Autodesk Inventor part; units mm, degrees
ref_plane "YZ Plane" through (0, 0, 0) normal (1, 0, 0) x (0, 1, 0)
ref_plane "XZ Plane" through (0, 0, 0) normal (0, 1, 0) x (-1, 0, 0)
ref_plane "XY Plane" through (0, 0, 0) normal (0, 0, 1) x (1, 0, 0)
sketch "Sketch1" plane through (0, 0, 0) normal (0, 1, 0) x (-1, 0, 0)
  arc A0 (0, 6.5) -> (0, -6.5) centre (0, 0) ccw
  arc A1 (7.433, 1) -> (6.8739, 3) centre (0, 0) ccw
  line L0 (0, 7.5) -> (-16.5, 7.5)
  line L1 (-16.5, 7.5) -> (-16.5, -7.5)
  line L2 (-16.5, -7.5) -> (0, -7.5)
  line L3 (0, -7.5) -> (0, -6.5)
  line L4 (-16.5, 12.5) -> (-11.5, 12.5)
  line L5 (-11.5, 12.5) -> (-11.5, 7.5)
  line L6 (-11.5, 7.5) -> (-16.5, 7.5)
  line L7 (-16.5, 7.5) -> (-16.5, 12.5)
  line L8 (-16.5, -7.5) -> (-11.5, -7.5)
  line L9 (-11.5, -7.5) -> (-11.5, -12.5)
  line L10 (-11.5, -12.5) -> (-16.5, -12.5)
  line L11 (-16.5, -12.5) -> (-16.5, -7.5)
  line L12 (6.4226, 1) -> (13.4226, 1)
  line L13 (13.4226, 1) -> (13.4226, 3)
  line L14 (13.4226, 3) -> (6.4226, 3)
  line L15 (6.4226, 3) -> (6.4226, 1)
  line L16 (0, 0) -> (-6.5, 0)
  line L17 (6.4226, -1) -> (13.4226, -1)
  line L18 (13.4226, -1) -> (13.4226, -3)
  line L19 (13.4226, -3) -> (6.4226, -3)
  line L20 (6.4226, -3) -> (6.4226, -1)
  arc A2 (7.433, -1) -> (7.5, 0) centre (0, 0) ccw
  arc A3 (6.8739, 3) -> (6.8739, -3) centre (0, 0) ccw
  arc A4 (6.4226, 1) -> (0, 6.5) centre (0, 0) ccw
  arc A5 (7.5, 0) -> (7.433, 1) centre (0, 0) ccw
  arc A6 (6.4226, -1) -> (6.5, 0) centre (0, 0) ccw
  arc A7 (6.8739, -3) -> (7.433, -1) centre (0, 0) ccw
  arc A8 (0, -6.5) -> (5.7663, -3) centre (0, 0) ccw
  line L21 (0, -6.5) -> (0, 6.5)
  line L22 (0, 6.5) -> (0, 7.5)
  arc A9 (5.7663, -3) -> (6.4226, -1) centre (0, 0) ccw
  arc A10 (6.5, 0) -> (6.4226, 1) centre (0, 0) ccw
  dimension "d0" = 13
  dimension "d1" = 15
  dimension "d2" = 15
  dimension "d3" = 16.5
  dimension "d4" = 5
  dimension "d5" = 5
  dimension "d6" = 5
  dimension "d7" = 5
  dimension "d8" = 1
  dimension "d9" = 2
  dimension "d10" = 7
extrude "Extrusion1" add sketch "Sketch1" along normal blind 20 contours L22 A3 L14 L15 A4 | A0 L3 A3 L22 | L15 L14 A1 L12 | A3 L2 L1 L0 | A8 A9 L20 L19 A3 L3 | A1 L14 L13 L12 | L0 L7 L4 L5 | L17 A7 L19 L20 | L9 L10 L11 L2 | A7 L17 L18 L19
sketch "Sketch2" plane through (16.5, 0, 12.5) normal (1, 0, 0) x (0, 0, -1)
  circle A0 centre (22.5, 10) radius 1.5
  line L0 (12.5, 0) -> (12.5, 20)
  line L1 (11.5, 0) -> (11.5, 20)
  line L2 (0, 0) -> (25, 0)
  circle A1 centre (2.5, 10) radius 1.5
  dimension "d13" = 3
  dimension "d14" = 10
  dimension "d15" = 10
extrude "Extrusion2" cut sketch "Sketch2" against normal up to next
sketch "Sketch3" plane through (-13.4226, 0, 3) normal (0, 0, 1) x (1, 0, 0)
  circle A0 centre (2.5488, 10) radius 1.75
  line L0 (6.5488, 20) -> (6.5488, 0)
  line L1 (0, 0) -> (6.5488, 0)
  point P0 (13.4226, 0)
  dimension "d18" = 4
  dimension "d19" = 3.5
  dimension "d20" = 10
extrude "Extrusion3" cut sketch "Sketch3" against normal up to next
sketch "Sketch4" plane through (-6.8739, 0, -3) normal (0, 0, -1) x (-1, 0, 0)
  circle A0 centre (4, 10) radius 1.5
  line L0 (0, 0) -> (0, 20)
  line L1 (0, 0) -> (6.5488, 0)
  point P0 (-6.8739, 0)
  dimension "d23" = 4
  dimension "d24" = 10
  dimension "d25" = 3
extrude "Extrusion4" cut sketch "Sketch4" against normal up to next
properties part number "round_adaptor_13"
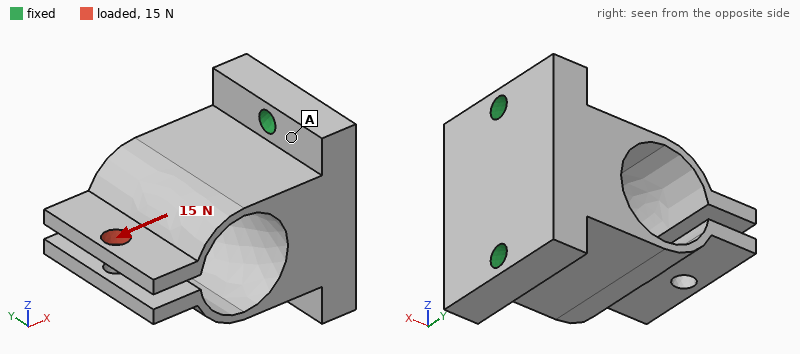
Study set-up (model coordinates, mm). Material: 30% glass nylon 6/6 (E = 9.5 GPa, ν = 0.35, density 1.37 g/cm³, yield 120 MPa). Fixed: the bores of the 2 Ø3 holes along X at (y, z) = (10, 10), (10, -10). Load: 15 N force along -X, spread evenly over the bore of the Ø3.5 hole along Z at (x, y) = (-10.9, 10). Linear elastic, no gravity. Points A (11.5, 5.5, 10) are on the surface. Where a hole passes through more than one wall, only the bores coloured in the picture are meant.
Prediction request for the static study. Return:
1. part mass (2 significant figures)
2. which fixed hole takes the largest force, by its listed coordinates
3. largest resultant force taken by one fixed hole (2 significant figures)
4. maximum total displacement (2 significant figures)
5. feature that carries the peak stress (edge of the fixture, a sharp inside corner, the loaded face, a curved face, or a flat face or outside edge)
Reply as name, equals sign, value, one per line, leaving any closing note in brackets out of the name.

part mass = 7.4 g
which fixed hole takes the largest force, by its listed coordinates = (10, 10)
largest resultant force taken by one fixed hole = 9.6 N
maximum total displacement = 0.42 mm
feature that carries the peak stress = a curved face
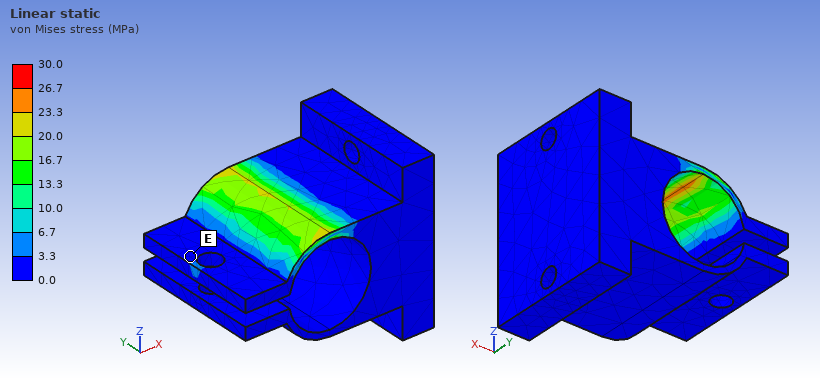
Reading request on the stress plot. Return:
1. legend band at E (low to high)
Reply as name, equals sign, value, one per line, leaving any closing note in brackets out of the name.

legend band at E = 0.0 to 3.3 MPa
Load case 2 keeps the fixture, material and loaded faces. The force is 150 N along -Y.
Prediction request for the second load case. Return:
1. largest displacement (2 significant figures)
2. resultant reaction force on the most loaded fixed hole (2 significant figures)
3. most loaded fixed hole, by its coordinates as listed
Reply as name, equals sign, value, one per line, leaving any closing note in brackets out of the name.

largest displacement = 0.47 mm
resultant reaction force on the most loaded fixed hole = 83 N
most loaded fixed hole, by its coordinates as listed = (10, 10)
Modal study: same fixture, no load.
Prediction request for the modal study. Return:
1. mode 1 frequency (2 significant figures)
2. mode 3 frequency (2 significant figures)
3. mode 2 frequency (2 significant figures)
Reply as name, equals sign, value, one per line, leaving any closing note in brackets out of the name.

mode 1 frequency = 1200 Hz
mode 3 frequency = 3000 Hz
mode 2 frequency = 1200 Hz
